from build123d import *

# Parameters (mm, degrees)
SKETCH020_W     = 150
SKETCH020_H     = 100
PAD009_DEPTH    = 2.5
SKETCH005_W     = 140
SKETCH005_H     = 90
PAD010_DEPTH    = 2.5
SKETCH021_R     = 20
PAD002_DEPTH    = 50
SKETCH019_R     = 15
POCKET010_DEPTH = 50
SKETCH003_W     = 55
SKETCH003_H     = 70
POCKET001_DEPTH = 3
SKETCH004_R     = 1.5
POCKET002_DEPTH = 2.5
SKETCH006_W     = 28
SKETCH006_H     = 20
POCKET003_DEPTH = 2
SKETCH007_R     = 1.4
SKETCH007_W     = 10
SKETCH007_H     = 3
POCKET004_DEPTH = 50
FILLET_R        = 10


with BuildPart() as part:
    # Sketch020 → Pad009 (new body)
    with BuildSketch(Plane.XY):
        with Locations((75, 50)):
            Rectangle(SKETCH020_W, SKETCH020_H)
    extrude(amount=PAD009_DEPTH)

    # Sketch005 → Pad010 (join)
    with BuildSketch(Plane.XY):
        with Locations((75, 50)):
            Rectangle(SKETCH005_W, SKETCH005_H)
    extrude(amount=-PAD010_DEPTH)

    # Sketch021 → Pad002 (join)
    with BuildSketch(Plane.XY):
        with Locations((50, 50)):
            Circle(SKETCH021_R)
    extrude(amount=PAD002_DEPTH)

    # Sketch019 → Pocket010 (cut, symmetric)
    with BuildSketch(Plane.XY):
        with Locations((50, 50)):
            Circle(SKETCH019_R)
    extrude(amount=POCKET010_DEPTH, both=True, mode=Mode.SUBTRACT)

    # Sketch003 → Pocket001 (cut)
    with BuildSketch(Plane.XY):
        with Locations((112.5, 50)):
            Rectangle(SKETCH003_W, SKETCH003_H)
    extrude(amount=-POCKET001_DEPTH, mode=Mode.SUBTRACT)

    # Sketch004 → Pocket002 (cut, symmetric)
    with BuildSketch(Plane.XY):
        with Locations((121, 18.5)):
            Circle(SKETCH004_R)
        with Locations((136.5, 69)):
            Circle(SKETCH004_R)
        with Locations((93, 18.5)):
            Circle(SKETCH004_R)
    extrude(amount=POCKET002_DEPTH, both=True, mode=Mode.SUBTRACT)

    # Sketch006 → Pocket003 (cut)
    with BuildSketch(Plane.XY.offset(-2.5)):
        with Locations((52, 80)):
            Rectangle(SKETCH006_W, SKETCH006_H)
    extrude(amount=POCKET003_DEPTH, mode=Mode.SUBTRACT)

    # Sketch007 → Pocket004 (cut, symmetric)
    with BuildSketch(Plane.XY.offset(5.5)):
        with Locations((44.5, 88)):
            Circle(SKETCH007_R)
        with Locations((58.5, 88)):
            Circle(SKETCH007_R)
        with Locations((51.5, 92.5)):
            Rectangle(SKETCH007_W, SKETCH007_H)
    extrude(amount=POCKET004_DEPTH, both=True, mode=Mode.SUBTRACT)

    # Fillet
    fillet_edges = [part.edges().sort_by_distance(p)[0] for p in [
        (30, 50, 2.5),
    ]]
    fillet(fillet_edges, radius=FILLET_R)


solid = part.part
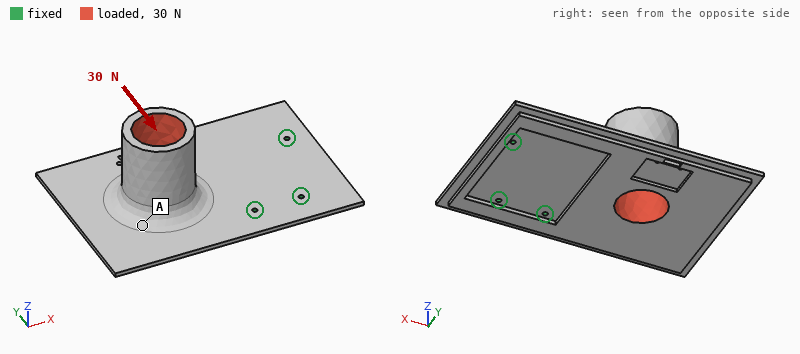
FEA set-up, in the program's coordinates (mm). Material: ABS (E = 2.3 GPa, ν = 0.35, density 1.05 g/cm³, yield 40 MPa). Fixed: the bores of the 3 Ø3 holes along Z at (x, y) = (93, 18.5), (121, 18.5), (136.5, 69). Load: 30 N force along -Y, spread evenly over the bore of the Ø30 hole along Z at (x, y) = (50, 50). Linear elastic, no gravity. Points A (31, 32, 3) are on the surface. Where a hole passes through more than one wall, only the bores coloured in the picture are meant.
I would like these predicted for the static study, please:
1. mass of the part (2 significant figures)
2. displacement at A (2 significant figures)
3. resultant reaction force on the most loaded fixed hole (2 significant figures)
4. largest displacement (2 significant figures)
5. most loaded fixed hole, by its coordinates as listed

88 g
0.60 mm
32 N
2.1 mm
(93, 18.5)
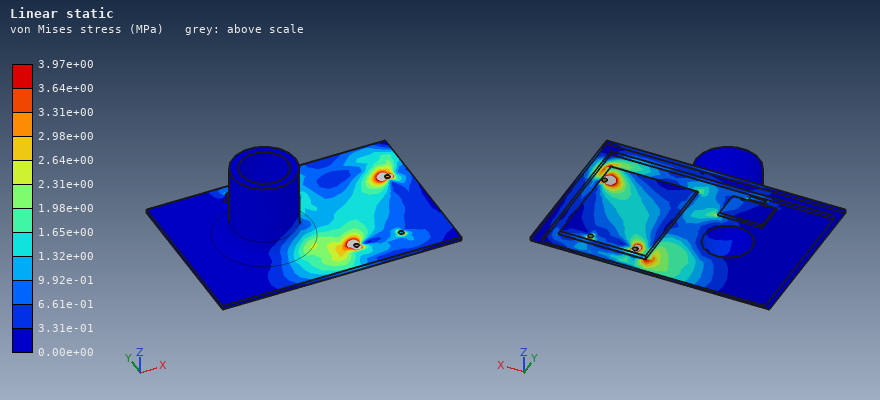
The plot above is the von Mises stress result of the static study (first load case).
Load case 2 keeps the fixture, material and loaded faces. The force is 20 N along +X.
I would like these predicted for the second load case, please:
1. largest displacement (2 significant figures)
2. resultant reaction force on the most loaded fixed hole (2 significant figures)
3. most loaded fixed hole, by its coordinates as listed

1.9 mm
20 N
(93, 18.5)
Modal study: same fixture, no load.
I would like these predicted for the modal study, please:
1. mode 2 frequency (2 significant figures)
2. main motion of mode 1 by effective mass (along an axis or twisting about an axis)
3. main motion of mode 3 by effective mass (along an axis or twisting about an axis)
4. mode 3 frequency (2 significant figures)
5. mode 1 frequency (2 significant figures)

160 Hz
along Z
along Z
460 Hz
52 Hz
